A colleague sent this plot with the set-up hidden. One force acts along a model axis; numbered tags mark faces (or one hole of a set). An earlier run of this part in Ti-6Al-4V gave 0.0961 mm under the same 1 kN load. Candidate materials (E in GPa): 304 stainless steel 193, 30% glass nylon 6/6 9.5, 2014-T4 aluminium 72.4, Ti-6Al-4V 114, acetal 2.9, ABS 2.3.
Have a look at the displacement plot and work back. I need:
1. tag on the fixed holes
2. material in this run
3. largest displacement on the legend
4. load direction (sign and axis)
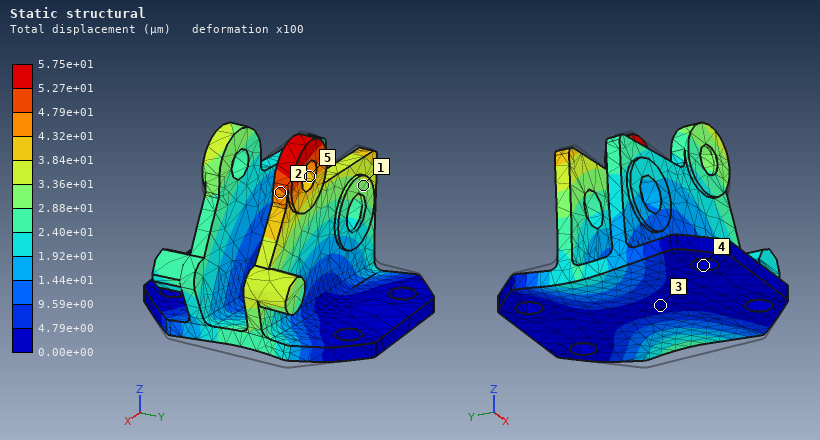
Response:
4
304 stainless steel
5.75e+01 µm
-X
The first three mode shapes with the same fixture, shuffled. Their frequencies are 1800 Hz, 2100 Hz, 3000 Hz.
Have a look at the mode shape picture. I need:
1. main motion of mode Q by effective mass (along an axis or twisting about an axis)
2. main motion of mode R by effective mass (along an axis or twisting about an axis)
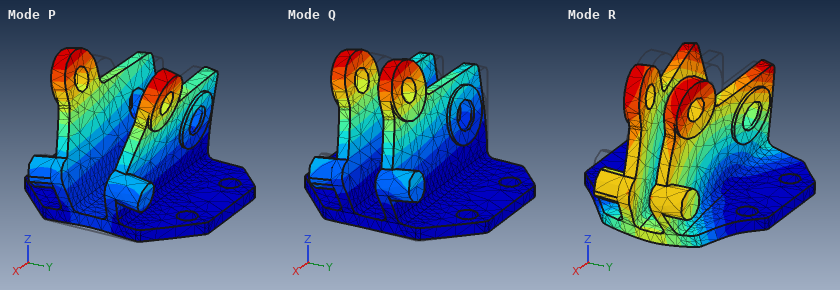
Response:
along Y
along X
